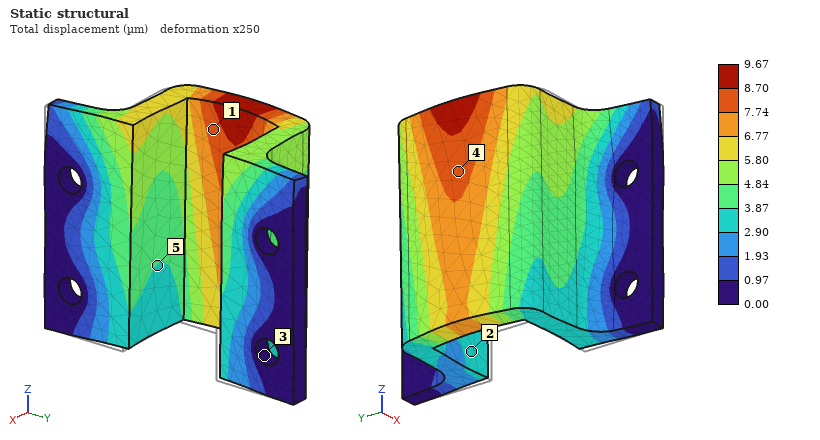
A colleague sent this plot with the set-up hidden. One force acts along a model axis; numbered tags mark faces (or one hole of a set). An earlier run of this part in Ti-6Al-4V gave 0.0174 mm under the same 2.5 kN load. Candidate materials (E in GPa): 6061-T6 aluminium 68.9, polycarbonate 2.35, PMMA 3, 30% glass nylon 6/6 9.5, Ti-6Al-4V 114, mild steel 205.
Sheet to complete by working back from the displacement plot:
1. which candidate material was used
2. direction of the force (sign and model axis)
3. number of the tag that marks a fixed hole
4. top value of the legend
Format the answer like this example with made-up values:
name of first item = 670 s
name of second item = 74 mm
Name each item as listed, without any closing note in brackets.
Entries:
which candidate material was used = mild steel
direction of the force = -X
number of the tag that marks a fixed hole = 3
top value of the legend = 9.67 µm
